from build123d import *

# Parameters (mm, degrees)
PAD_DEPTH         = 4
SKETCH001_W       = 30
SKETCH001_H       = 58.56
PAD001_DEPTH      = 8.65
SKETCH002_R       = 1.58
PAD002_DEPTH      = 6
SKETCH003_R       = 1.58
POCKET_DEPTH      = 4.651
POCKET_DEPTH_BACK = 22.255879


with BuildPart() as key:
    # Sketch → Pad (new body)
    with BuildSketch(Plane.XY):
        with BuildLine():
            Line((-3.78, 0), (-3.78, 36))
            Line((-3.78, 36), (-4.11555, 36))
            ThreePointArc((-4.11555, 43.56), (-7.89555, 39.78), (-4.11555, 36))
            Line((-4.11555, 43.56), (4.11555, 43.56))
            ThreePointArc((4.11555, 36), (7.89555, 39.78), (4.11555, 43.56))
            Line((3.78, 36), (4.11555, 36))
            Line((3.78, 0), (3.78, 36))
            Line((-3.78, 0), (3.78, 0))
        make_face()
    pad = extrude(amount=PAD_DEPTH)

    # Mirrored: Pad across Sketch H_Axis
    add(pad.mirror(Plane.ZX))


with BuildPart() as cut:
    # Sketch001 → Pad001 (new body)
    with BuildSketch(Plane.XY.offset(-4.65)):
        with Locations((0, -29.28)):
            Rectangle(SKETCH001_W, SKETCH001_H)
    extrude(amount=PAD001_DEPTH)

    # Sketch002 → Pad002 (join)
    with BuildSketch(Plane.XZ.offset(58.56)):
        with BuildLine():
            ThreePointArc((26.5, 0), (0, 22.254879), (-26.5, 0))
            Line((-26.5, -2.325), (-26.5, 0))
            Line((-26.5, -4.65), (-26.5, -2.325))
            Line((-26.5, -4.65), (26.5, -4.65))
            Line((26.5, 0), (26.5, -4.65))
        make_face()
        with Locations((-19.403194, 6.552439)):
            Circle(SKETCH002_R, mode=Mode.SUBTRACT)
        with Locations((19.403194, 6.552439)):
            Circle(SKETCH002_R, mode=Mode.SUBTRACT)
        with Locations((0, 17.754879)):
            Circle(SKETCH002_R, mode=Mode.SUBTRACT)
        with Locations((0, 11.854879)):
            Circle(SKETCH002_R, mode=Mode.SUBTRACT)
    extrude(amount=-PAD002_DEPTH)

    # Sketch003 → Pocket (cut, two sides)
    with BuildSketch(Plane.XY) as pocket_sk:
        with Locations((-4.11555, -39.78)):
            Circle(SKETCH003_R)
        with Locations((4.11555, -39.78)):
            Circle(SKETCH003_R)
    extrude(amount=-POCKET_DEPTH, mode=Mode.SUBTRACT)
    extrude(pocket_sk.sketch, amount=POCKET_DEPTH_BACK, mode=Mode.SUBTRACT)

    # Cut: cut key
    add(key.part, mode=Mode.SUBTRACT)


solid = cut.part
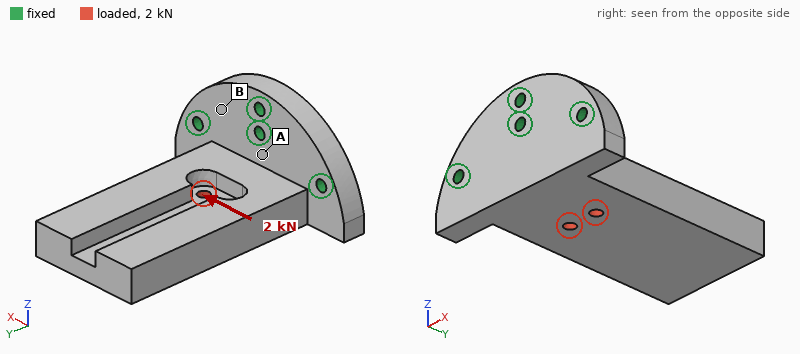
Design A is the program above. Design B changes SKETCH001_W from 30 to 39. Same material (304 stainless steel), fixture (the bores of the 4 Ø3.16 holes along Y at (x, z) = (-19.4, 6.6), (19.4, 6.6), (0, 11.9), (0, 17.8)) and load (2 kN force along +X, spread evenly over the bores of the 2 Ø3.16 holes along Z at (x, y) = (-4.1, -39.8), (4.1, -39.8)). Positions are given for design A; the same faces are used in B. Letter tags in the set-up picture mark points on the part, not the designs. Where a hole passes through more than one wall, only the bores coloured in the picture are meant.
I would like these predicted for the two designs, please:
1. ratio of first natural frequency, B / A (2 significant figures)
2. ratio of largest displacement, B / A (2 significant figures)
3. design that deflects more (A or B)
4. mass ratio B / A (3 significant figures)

0.98
0.52
A
1.22
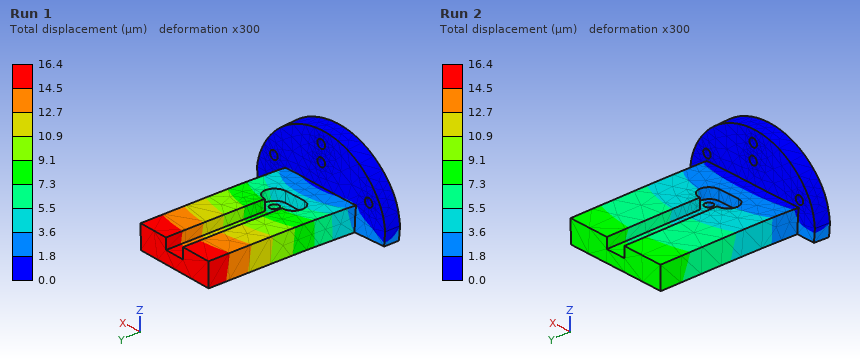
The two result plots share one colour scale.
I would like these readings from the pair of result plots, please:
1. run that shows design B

Run 2
